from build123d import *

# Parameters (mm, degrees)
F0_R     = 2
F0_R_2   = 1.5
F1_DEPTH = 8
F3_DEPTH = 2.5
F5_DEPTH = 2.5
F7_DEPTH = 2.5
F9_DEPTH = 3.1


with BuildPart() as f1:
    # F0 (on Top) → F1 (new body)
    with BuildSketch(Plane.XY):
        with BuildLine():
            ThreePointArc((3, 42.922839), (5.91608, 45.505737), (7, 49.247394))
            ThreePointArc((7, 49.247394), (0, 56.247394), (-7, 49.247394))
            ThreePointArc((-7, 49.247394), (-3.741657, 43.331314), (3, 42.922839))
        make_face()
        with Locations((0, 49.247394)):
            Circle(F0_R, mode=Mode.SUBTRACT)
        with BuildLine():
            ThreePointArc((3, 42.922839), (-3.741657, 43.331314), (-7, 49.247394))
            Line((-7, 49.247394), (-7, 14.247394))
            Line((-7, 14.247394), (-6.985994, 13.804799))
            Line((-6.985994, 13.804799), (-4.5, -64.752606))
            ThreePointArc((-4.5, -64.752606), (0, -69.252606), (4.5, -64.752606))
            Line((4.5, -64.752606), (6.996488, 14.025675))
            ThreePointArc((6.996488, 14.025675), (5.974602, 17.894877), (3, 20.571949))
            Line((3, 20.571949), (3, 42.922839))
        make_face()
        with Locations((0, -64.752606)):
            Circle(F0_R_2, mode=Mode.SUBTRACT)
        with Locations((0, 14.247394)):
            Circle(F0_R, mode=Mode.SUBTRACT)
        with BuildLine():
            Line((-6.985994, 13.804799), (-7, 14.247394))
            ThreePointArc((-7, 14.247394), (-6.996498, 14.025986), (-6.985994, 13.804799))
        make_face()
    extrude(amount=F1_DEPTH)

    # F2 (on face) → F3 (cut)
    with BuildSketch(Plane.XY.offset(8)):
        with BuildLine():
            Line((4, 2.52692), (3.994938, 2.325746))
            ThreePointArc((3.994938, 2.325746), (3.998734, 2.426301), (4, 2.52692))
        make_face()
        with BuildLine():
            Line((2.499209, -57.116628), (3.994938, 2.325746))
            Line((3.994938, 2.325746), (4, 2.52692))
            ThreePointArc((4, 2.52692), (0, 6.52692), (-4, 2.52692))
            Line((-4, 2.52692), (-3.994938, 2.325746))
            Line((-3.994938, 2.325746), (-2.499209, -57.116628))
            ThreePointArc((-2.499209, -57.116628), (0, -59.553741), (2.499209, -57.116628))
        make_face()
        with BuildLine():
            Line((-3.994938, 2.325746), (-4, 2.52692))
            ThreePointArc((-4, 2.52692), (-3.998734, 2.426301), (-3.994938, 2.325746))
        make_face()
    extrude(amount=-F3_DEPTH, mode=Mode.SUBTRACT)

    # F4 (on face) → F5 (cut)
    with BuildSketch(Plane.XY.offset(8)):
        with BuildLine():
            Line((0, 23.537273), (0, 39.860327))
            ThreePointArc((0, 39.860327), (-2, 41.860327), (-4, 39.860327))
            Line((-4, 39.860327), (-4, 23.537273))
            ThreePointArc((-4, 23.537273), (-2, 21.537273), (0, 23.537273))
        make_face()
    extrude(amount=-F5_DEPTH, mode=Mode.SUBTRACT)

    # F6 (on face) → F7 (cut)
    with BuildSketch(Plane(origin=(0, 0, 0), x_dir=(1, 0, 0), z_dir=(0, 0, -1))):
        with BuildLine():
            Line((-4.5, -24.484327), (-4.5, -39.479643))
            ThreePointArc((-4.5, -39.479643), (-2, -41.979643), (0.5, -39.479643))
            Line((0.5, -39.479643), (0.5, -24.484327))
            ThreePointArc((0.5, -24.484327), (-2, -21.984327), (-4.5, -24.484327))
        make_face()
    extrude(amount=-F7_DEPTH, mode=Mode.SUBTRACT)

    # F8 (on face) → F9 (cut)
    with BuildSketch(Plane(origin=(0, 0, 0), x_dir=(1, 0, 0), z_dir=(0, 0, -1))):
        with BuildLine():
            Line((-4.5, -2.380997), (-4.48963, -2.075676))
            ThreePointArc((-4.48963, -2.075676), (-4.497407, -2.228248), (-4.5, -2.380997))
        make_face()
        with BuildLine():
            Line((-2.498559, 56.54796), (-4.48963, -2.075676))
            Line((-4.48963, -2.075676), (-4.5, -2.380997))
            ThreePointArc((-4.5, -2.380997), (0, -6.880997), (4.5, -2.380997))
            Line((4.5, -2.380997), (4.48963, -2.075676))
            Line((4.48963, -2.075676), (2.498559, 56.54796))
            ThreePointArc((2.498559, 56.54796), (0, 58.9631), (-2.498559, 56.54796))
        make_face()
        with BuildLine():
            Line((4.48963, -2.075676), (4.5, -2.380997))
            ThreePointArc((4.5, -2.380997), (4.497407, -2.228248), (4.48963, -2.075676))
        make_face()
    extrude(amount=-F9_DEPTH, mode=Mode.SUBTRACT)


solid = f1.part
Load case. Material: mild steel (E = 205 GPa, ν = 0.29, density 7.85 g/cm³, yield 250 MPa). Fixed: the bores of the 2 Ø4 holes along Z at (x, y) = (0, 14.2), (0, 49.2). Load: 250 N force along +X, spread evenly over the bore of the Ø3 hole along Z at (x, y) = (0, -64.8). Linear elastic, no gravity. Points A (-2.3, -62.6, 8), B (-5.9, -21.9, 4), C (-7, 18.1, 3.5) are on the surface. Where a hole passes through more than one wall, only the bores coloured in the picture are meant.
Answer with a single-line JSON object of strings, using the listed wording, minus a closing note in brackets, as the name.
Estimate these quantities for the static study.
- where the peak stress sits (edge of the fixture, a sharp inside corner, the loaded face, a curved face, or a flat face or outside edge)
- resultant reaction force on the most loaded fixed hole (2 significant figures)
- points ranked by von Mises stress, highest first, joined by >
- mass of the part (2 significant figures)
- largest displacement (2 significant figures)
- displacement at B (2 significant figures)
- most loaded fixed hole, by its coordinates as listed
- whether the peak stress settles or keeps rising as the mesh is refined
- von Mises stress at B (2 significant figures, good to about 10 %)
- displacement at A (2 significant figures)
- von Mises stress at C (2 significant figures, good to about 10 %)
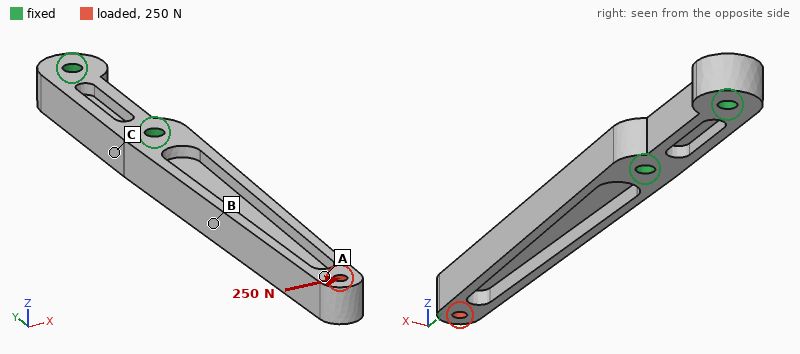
{"where the peak stress sits": "edge of the fixture", "resultant reaction force on the most loaded fixed hole": "510 N", "points ranked by von Mises stress, highest first, joined by >": "B > C > A", "mass of the part": "63 g", "largest displacement": "0.23 mm", "displacement at B": "0.057 mm", "most loaded fixed hole, by its coordinates as listed": "(0, 14.2)", "whether the peak stress settles or keeps rising as the mesh is refined": "keeps rising", "von Mises stress at B": "70 MPa", "displacement at A": "0.20 mm", "von Mises stress at C": "34 MPa"}
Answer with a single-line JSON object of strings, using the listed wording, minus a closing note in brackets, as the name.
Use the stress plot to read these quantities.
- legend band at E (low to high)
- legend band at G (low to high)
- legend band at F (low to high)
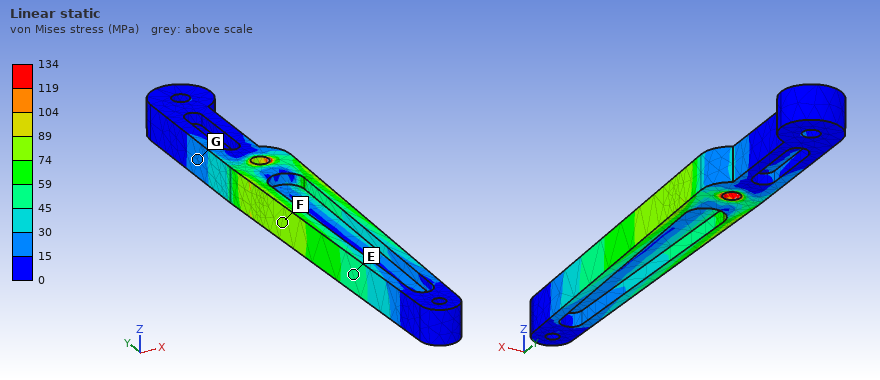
{"legend band at E": "45 to 59 MPa", "legend band at G": "15 to 30 MPa", "legend band at F": "74 to 89 MPa"}
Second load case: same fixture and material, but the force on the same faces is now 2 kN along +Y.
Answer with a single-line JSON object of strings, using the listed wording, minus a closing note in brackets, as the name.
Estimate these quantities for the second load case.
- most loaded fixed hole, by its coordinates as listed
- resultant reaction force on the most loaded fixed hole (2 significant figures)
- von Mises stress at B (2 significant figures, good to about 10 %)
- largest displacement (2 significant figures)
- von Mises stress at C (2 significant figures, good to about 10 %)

{"most loaded fixed hole, by its coordinates as listed": "(0, 14.2)", "resultant reaction force on the most loaded fixed hole": "1.9 kN", "von Mises stress at B": "37 MPa", "largest displacement": "30 µm", "von Mises stress at C": "6.2 MPa"}
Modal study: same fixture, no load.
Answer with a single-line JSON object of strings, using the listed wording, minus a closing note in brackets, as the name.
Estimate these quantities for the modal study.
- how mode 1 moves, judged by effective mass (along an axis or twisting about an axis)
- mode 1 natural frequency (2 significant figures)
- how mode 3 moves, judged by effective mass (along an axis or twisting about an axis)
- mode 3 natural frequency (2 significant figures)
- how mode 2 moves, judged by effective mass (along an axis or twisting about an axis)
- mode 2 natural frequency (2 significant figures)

{"how mode 1 moves, judged by effective mass": "along Z", "mode 1 natural frequency": "890 Hz", "how mode 3 moves, judged by effective mass": "twisting about Y", "mode 3 natural frequency": "4400 Hz", "how mode 2 moves, judged by effective mass": "along X", "mode 2 natural frequency": "1700 Hz"}
